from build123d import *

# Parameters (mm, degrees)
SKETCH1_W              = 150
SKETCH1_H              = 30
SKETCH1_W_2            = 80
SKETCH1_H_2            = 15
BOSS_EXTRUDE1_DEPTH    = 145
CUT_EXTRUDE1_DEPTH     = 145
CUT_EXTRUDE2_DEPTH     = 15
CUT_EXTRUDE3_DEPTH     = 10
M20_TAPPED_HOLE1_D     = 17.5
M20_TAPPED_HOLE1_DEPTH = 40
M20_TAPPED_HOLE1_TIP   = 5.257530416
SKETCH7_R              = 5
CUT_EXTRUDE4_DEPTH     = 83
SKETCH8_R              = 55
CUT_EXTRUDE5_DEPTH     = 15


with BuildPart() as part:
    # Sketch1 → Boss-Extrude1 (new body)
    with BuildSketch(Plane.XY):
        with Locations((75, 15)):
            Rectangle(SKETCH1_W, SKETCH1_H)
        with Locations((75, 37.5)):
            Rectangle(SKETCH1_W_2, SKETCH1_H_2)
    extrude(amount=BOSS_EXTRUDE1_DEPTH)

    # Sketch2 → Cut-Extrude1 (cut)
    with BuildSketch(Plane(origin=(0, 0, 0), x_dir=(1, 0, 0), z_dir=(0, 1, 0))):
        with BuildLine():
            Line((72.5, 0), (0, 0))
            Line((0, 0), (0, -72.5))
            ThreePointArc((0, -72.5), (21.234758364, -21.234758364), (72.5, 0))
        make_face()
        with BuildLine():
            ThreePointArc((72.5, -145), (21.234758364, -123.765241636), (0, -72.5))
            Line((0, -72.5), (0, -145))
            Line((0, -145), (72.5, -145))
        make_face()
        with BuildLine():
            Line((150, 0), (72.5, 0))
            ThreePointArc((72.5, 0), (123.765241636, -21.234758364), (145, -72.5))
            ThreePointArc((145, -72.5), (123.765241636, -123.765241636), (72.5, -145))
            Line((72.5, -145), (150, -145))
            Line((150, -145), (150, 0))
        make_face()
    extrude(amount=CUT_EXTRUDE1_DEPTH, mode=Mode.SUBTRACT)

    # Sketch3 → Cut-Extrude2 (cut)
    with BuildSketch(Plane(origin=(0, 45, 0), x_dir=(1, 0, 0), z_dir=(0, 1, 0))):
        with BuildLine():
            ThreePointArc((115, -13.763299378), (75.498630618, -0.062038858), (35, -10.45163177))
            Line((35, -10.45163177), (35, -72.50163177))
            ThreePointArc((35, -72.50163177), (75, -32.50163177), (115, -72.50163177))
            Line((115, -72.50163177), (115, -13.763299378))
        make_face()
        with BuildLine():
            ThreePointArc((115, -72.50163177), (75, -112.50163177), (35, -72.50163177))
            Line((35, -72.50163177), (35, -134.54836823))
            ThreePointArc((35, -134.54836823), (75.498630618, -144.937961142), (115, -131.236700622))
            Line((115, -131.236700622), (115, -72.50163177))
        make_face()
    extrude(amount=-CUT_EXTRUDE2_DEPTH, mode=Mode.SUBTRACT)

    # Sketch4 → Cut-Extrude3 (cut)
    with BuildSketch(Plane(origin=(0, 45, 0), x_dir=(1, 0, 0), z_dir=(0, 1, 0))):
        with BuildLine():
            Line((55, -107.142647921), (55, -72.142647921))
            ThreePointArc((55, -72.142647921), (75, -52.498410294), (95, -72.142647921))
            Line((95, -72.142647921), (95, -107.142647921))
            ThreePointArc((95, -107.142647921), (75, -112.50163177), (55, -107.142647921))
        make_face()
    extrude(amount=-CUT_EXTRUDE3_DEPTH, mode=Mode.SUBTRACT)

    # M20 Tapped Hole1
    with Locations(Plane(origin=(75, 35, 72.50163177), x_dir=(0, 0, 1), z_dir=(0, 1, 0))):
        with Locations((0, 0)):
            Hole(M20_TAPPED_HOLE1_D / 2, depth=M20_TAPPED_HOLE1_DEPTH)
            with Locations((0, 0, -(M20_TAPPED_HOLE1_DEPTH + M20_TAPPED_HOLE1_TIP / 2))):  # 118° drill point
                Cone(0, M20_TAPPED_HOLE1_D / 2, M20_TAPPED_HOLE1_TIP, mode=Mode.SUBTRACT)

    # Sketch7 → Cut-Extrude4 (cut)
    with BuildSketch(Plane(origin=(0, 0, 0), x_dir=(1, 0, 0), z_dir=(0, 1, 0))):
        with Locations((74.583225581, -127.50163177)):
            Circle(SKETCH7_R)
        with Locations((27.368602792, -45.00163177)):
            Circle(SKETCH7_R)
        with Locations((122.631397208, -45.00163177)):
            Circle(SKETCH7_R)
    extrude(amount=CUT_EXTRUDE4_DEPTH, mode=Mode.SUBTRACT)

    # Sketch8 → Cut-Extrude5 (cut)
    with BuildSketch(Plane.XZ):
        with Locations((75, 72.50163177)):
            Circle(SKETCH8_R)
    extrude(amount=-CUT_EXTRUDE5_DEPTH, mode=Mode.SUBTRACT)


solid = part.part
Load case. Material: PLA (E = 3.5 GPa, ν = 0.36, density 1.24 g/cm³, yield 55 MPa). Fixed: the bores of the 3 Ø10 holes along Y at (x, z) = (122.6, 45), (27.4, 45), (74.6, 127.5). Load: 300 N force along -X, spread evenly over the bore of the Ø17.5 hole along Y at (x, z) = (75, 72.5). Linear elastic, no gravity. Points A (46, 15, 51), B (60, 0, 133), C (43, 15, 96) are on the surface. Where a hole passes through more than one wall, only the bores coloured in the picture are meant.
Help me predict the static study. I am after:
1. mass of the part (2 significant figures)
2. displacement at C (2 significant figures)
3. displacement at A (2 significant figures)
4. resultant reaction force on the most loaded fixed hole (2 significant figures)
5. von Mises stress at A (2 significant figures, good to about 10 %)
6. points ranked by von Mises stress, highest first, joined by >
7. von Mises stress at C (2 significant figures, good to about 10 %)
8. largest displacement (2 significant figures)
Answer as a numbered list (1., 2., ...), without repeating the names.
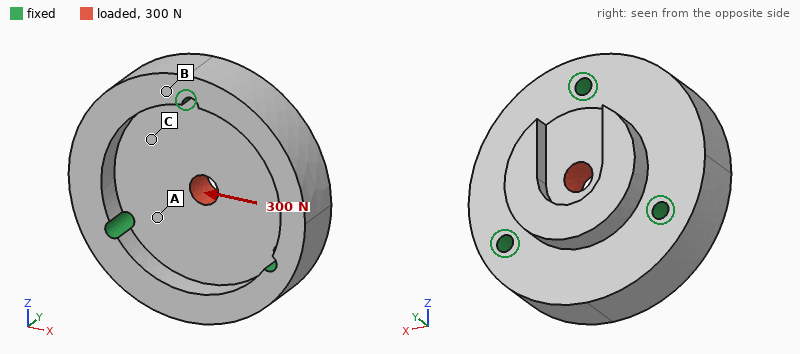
1. 490 g
2. 1.8 µm
3. 1.0 µm
4. 110 N
5. 0.19 MPa
6. A > C > B
7. 0.100 MPa
8. 3.5 µm
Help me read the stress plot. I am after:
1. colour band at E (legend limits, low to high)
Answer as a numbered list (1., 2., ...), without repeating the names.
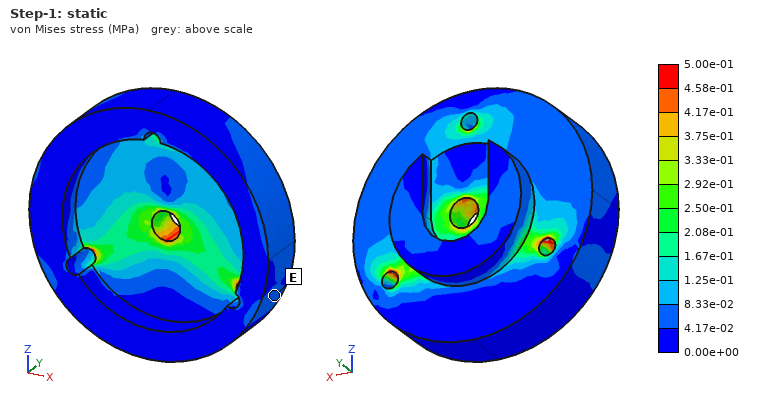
1. 4.17e-02 to 8.33e-02 MPa
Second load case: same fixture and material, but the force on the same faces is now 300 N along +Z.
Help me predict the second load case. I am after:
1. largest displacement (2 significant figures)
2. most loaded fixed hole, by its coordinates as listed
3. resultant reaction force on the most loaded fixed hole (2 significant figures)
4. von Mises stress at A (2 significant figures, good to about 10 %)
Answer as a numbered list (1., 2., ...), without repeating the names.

1. 3.7 µm
2. (74.6, 127.5)
3. 110 N
4. 0.13 MPa
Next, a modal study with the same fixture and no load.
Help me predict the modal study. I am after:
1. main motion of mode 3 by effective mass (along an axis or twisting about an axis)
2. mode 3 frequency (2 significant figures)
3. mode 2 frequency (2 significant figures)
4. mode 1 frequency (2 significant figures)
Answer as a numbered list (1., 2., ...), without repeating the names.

1. along Y
2. 2300 Hz
3. 2100 Hz
4. 2000 Hz
